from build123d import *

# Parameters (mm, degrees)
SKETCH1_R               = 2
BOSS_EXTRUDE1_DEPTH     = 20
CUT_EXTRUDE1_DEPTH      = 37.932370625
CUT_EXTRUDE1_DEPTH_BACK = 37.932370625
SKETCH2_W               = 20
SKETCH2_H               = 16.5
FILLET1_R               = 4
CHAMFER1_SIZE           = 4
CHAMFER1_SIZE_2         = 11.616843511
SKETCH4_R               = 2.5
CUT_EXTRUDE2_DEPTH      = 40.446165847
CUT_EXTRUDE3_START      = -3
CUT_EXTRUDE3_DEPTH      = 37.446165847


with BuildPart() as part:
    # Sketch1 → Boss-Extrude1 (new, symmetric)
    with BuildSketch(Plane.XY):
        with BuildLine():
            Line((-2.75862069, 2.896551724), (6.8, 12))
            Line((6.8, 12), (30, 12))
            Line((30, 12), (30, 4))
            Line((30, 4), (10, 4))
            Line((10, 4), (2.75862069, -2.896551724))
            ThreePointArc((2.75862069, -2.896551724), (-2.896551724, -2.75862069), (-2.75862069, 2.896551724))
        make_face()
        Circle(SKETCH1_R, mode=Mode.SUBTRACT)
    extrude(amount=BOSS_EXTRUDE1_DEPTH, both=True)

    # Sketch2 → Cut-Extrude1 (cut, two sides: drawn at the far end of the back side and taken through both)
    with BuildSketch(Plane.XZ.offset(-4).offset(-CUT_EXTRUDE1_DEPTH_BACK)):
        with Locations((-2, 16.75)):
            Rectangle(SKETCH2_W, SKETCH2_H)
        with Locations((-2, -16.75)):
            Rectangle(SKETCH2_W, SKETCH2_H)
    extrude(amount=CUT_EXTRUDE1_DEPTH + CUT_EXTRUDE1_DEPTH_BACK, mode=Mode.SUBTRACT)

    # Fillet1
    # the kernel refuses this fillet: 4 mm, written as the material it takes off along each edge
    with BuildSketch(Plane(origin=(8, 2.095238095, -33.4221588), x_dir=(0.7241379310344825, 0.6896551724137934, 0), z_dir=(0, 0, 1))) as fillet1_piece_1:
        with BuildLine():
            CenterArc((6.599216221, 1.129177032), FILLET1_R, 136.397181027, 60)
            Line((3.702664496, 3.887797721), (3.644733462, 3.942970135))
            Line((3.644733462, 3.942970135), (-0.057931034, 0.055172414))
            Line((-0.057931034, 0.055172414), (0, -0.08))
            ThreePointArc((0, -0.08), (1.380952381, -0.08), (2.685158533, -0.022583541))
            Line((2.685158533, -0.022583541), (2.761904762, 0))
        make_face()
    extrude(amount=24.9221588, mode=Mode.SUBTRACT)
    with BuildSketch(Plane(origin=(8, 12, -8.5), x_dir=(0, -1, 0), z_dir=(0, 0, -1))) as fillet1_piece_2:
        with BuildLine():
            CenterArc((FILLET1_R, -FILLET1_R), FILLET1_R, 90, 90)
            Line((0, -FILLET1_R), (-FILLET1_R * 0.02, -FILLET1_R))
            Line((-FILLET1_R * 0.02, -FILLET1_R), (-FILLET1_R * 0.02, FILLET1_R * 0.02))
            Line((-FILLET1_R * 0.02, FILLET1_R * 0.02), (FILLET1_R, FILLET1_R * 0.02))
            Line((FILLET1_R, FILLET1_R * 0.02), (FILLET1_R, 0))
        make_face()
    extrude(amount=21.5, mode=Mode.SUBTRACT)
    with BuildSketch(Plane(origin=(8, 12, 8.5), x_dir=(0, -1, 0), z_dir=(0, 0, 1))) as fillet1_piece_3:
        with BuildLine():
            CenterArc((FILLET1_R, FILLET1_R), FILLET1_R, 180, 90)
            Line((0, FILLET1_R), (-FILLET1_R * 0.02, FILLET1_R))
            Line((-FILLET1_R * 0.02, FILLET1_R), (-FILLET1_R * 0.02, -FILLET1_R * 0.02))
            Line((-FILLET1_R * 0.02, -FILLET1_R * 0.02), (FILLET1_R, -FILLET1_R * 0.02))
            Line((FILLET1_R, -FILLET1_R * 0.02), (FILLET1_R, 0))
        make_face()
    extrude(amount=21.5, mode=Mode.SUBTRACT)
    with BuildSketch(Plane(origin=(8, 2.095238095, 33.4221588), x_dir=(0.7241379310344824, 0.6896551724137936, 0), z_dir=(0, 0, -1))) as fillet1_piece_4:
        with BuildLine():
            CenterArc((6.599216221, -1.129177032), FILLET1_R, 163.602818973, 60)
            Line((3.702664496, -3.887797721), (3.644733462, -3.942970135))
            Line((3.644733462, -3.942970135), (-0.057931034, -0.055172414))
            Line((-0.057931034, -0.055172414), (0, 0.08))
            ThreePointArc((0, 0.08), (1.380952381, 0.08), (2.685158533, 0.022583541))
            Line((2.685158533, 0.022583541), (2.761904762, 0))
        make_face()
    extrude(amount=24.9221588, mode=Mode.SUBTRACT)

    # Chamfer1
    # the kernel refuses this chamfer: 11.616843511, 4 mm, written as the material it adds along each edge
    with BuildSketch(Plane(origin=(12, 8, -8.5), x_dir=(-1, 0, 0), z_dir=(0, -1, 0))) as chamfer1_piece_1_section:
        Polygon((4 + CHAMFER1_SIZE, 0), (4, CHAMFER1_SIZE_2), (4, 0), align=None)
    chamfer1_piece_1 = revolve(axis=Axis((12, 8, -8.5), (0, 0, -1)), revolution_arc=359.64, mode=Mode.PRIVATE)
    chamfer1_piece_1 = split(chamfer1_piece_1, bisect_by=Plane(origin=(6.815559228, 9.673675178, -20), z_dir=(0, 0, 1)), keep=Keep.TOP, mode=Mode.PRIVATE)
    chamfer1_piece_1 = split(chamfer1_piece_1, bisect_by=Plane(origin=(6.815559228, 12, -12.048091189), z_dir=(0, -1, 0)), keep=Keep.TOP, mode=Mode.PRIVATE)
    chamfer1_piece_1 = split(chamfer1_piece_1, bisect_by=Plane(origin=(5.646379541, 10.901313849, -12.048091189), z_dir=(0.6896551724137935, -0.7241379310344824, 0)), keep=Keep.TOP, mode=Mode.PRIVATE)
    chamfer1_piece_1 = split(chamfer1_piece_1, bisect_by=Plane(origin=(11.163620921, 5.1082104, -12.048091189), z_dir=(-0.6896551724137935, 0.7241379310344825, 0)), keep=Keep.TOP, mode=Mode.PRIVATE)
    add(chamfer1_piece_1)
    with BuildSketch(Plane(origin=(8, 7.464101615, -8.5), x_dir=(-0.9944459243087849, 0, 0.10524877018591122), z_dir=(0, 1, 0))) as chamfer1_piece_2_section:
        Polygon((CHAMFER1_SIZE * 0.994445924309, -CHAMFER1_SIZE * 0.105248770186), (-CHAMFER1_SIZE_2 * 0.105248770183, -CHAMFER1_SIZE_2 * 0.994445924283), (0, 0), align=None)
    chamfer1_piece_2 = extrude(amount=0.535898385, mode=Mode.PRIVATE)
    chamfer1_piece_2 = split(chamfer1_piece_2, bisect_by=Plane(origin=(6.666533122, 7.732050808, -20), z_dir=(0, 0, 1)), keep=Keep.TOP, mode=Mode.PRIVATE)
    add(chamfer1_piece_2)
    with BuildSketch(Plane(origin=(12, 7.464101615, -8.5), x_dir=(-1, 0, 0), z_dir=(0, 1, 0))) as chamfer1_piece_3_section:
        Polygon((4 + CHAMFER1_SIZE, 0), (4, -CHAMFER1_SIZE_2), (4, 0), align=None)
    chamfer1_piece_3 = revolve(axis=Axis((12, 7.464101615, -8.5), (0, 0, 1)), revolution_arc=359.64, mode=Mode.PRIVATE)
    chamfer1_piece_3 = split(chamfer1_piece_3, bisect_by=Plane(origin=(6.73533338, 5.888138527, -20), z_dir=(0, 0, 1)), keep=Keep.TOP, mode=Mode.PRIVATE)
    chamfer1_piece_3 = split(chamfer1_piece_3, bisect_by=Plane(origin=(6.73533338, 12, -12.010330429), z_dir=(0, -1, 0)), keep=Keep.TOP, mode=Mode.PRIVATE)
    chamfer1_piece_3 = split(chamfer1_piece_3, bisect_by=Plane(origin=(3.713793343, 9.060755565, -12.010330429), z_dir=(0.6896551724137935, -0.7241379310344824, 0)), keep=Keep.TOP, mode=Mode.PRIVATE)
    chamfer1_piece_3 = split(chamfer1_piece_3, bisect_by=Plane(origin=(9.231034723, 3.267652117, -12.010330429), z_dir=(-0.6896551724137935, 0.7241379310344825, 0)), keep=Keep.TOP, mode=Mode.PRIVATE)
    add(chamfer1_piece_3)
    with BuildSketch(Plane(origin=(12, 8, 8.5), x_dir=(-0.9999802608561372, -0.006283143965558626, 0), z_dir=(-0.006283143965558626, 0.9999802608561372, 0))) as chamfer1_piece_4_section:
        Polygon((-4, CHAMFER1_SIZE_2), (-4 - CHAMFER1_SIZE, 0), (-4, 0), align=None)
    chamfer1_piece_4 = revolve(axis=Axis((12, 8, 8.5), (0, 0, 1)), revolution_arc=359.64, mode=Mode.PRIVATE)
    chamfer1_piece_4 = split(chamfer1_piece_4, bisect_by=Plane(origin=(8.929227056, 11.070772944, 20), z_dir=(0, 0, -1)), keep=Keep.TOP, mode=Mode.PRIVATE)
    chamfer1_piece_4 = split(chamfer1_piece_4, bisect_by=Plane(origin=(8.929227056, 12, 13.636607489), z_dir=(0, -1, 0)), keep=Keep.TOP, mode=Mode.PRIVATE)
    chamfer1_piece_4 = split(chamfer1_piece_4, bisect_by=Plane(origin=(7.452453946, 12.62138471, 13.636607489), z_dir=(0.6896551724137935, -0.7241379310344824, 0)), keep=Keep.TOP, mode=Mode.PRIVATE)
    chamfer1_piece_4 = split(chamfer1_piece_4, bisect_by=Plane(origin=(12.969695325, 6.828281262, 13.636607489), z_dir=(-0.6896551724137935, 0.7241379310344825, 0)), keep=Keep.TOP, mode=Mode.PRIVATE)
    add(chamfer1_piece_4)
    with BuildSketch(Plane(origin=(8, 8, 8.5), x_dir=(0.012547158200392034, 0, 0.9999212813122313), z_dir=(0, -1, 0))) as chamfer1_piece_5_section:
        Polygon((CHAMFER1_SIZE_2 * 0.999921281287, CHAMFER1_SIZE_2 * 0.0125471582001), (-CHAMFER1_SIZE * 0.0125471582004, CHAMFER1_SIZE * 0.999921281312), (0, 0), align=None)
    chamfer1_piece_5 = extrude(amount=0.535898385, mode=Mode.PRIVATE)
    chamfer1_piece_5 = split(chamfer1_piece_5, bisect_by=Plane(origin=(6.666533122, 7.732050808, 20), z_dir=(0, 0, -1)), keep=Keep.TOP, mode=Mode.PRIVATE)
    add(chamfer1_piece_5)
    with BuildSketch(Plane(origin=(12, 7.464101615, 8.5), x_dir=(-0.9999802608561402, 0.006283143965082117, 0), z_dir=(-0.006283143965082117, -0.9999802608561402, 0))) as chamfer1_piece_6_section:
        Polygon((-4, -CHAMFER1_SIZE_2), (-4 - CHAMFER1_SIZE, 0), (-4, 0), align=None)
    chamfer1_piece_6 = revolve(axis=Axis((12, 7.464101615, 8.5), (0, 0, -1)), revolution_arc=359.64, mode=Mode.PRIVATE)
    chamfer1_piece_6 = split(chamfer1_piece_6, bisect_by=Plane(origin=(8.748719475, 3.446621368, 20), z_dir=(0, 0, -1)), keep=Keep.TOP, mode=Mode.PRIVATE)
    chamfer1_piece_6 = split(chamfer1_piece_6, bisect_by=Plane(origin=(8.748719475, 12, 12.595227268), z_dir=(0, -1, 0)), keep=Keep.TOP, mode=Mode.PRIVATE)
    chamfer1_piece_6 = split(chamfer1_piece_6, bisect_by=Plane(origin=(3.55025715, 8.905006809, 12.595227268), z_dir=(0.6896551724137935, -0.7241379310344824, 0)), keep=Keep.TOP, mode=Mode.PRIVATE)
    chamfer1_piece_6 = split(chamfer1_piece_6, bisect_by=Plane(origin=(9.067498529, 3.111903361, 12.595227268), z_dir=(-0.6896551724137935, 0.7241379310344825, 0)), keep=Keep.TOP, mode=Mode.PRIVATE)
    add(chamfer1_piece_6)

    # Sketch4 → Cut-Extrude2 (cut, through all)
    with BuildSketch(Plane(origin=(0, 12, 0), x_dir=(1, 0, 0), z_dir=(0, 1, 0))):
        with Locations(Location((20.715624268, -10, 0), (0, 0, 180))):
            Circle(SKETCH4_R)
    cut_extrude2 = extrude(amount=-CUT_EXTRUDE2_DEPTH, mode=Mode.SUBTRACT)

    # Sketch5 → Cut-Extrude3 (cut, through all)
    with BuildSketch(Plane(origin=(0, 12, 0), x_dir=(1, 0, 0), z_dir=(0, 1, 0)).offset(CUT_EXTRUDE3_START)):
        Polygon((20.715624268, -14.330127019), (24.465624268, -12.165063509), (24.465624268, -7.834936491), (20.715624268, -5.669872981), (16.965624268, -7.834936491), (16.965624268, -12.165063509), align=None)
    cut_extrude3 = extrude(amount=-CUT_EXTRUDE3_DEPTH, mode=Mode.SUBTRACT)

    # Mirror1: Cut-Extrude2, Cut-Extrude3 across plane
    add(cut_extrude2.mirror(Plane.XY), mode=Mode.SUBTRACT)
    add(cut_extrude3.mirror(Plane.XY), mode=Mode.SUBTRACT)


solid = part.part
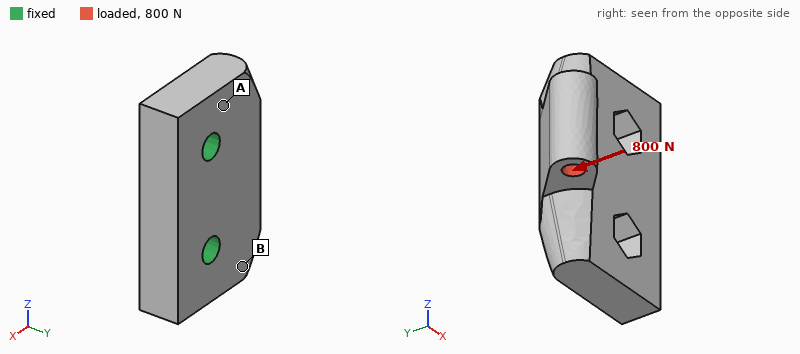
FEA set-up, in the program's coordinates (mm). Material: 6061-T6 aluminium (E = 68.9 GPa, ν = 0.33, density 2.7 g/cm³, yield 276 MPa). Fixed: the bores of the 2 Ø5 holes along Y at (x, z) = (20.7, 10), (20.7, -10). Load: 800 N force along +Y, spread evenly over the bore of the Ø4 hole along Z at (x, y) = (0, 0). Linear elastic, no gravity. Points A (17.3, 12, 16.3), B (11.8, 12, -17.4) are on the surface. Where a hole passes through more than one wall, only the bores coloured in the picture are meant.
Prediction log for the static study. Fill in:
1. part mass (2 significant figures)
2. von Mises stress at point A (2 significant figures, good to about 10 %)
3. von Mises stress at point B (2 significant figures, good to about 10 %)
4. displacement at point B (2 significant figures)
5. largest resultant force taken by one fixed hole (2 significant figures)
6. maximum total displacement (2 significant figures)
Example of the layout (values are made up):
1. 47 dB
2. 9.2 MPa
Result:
1. 23 g
2. 33 MPa
3. 19 MPa
4. 0.023 mm
5. 440 N
6. 0.11 mm
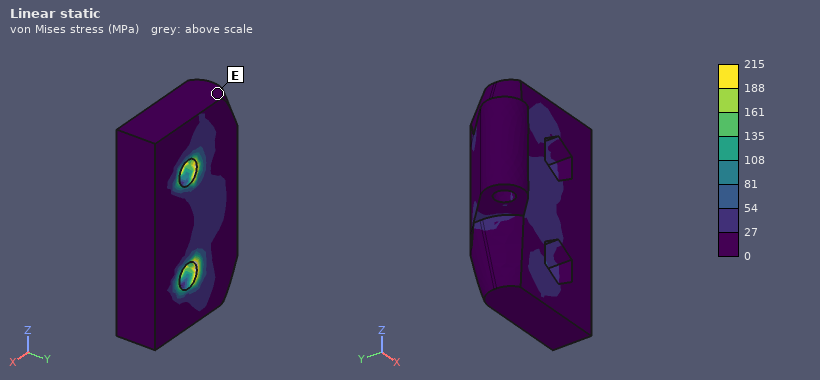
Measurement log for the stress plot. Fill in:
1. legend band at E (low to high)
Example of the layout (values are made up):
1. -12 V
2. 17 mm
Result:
1. 0 to 27 MPa
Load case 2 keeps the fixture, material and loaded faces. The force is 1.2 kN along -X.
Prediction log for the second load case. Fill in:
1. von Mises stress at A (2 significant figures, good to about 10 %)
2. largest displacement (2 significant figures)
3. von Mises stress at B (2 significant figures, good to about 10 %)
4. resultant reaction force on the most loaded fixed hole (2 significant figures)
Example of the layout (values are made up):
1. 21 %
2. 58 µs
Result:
1. 24 MPa
2. 93 µm
3. 16 MPa
4. 600 N
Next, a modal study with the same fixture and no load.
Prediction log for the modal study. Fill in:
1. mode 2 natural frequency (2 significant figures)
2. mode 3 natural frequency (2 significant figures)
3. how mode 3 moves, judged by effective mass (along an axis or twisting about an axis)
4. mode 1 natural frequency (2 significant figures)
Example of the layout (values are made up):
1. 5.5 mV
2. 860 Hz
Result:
1. 19 kHz
2. 21 kHz
3. along Z
4. 6800 Hz
